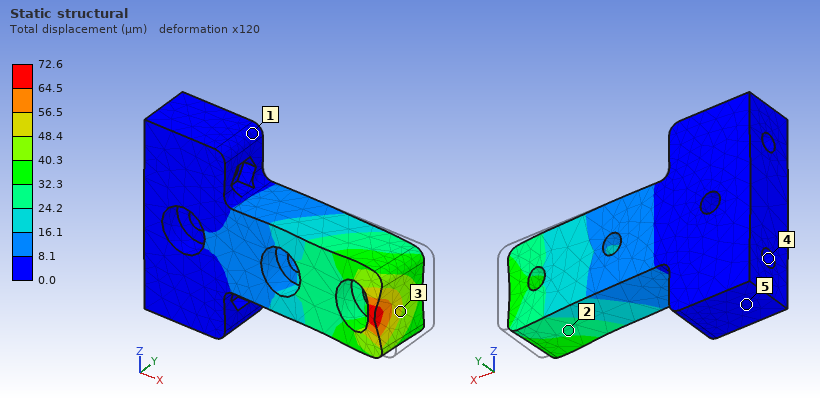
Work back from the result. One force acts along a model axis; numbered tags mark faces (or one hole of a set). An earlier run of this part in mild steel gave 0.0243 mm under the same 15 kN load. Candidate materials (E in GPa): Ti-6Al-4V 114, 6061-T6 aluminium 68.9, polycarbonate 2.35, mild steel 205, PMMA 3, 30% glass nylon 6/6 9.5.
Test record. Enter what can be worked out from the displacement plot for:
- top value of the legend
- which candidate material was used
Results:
72.6 µm
6061-T6 aluminium
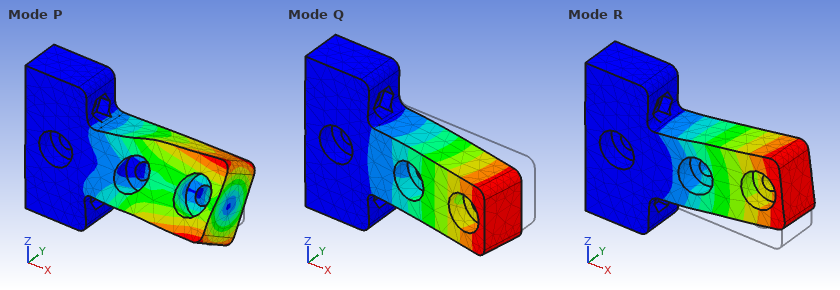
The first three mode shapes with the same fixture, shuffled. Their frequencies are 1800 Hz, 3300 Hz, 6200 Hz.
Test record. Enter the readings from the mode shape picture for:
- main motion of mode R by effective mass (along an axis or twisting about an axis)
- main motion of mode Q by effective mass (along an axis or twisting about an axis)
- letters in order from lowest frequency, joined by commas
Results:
along Z
along Y
Q, R, P
